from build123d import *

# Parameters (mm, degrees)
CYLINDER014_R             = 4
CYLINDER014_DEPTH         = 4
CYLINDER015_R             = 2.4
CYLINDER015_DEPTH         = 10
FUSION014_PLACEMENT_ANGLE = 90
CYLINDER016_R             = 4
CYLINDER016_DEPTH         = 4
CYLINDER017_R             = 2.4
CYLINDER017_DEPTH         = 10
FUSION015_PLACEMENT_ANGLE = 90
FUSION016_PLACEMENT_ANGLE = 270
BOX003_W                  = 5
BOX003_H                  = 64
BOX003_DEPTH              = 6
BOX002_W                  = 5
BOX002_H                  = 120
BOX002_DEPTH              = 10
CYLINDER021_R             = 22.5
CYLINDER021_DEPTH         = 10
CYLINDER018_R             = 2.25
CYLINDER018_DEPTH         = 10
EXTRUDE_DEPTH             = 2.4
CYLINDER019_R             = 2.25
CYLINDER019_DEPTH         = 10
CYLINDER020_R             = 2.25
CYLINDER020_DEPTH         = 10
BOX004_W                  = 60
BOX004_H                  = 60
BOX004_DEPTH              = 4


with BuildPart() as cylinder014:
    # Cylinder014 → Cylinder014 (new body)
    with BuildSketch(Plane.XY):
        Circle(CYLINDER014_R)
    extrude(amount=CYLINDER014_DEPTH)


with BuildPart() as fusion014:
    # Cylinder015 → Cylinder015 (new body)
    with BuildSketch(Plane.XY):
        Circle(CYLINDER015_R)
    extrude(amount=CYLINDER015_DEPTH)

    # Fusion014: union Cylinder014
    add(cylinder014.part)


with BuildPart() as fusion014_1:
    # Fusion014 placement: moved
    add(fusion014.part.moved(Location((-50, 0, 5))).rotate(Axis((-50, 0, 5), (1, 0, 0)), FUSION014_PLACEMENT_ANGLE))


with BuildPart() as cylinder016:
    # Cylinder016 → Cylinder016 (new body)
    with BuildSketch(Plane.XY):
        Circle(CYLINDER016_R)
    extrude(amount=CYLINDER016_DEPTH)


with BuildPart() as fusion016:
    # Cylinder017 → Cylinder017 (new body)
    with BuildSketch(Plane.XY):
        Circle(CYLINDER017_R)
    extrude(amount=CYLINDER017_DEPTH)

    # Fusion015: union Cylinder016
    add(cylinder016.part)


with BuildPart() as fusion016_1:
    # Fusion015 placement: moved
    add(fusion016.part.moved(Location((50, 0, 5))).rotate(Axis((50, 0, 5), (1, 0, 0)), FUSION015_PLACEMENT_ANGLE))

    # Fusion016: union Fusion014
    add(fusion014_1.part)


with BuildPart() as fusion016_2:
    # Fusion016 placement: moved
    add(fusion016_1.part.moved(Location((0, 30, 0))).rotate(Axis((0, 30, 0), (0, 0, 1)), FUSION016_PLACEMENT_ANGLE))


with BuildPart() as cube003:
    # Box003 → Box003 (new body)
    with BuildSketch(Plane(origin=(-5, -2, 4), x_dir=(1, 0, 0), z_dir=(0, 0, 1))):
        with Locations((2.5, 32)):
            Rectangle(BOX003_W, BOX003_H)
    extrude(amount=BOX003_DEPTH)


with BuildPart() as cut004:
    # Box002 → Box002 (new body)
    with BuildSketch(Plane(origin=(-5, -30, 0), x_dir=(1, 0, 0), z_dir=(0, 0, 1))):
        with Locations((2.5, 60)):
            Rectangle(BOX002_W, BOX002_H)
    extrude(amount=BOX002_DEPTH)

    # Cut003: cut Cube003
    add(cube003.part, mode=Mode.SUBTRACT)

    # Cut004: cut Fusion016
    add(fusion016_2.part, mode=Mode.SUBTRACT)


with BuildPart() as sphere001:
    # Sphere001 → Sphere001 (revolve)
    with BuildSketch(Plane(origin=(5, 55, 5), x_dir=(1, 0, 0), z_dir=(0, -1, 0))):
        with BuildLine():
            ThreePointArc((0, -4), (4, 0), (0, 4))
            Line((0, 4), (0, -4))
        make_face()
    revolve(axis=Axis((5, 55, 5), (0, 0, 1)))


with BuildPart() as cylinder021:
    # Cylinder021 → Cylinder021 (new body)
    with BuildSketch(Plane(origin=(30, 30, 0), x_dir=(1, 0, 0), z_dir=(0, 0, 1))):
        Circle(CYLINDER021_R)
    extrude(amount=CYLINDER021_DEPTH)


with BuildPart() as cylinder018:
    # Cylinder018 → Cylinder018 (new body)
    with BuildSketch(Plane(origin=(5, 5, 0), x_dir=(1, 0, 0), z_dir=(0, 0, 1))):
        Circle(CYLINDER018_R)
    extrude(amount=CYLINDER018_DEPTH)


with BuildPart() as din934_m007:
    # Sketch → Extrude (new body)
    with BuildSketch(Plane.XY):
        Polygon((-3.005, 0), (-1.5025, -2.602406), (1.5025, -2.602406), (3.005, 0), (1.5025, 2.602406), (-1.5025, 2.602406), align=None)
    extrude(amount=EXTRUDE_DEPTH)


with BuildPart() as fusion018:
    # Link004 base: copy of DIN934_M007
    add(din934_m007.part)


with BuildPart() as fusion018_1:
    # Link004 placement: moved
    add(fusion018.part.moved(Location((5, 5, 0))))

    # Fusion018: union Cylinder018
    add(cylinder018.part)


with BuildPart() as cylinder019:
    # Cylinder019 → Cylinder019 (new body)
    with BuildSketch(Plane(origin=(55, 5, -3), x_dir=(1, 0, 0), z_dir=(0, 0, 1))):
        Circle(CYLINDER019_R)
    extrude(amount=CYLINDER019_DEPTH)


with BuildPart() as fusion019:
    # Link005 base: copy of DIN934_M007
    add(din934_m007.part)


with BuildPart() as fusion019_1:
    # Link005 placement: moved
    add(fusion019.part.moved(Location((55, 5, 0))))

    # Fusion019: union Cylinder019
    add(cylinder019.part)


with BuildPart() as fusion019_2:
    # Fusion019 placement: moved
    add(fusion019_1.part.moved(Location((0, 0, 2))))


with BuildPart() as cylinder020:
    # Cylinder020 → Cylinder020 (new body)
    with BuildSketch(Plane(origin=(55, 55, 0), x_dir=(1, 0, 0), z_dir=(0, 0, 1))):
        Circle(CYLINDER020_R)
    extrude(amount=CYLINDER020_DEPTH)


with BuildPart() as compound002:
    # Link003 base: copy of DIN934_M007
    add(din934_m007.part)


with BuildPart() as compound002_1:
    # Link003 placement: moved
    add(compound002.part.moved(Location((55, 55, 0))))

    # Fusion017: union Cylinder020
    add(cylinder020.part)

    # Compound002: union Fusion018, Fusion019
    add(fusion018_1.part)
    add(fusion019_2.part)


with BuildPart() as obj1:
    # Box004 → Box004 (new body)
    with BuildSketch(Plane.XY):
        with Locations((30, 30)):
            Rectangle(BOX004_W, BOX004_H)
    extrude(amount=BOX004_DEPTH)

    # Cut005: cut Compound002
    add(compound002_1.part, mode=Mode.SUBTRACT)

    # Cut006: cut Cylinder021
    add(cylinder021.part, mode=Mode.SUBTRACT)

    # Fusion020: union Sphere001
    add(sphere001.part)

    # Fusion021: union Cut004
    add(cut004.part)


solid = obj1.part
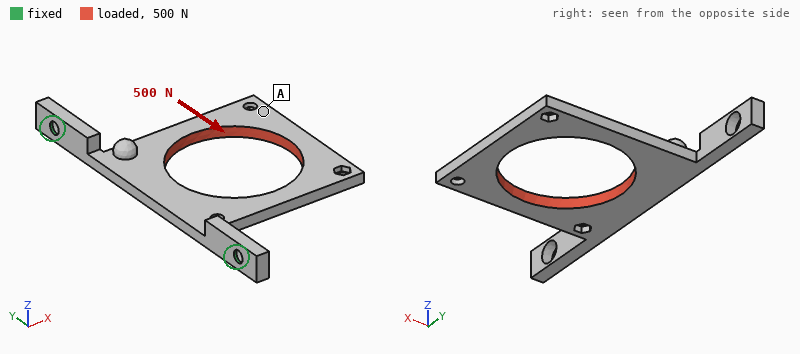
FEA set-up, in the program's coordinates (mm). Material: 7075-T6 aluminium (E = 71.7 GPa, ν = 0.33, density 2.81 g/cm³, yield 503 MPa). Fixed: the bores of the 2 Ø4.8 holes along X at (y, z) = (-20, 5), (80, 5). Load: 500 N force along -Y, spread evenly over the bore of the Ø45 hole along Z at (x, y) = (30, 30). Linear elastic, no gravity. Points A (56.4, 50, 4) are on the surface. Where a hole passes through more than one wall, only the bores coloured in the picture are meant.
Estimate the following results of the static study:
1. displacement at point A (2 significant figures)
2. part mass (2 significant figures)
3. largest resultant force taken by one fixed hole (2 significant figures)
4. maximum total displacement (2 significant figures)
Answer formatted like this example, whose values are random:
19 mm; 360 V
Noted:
0.17 mm; 33 g; 320 N; 0.18 mm
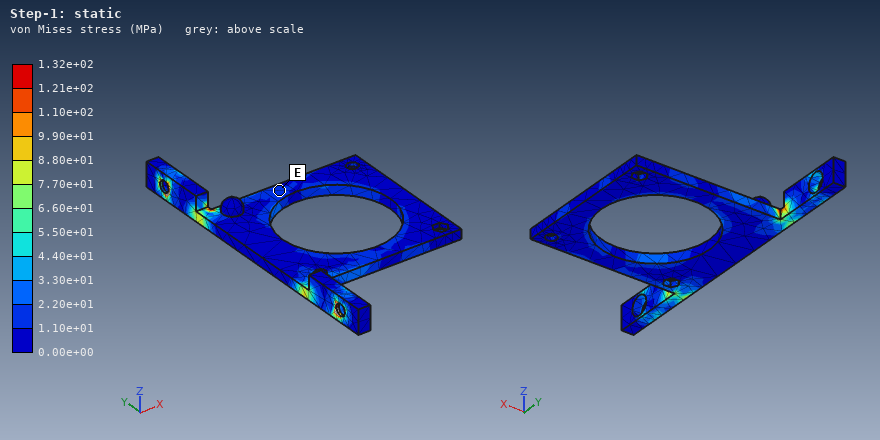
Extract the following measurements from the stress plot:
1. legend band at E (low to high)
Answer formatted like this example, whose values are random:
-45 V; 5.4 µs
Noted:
1.10e+01 to 2.20e+01 MPa
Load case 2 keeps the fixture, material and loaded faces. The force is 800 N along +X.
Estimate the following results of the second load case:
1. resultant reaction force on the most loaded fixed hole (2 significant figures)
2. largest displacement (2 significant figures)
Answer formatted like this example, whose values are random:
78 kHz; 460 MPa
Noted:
840 N; 0.39 mm
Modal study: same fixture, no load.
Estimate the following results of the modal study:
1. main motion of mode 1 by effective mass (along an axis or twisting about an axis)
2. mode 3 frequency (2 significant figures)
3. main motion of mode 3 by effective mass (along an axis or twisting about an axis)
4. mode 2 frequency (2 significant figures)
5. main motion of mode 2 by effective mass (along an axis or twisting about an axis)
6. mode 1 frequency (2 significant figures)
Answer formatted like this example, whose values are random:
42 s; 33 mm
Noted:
along Z; 1900 Hz; along Y; 1400 Hz; twisting about X; 370 Hz
